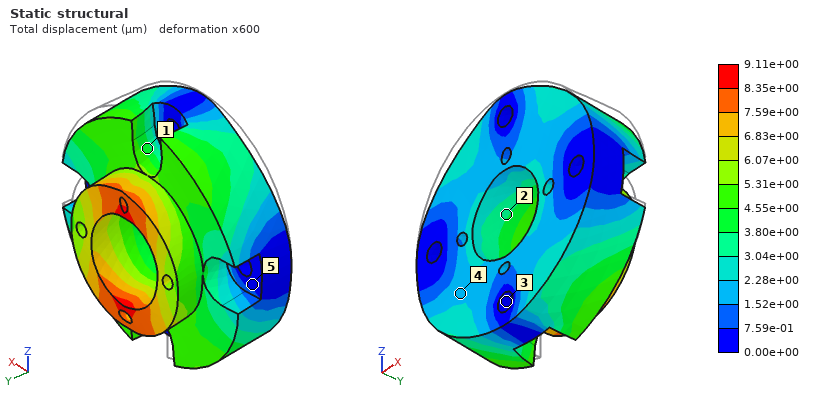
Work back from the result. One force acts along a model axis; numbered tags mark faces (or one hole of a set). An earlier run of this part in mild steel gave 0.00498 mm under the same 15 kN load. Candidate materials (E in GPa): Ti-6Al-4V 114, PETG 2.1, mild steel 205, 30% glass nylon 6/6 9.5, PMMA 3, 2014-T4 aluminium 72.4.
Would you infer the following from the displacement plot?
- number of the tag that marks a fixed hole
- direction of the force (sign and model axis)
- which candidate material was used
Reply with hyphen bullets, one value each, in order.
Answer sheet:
- 3
- -Z
- Ti-6Al-4V
